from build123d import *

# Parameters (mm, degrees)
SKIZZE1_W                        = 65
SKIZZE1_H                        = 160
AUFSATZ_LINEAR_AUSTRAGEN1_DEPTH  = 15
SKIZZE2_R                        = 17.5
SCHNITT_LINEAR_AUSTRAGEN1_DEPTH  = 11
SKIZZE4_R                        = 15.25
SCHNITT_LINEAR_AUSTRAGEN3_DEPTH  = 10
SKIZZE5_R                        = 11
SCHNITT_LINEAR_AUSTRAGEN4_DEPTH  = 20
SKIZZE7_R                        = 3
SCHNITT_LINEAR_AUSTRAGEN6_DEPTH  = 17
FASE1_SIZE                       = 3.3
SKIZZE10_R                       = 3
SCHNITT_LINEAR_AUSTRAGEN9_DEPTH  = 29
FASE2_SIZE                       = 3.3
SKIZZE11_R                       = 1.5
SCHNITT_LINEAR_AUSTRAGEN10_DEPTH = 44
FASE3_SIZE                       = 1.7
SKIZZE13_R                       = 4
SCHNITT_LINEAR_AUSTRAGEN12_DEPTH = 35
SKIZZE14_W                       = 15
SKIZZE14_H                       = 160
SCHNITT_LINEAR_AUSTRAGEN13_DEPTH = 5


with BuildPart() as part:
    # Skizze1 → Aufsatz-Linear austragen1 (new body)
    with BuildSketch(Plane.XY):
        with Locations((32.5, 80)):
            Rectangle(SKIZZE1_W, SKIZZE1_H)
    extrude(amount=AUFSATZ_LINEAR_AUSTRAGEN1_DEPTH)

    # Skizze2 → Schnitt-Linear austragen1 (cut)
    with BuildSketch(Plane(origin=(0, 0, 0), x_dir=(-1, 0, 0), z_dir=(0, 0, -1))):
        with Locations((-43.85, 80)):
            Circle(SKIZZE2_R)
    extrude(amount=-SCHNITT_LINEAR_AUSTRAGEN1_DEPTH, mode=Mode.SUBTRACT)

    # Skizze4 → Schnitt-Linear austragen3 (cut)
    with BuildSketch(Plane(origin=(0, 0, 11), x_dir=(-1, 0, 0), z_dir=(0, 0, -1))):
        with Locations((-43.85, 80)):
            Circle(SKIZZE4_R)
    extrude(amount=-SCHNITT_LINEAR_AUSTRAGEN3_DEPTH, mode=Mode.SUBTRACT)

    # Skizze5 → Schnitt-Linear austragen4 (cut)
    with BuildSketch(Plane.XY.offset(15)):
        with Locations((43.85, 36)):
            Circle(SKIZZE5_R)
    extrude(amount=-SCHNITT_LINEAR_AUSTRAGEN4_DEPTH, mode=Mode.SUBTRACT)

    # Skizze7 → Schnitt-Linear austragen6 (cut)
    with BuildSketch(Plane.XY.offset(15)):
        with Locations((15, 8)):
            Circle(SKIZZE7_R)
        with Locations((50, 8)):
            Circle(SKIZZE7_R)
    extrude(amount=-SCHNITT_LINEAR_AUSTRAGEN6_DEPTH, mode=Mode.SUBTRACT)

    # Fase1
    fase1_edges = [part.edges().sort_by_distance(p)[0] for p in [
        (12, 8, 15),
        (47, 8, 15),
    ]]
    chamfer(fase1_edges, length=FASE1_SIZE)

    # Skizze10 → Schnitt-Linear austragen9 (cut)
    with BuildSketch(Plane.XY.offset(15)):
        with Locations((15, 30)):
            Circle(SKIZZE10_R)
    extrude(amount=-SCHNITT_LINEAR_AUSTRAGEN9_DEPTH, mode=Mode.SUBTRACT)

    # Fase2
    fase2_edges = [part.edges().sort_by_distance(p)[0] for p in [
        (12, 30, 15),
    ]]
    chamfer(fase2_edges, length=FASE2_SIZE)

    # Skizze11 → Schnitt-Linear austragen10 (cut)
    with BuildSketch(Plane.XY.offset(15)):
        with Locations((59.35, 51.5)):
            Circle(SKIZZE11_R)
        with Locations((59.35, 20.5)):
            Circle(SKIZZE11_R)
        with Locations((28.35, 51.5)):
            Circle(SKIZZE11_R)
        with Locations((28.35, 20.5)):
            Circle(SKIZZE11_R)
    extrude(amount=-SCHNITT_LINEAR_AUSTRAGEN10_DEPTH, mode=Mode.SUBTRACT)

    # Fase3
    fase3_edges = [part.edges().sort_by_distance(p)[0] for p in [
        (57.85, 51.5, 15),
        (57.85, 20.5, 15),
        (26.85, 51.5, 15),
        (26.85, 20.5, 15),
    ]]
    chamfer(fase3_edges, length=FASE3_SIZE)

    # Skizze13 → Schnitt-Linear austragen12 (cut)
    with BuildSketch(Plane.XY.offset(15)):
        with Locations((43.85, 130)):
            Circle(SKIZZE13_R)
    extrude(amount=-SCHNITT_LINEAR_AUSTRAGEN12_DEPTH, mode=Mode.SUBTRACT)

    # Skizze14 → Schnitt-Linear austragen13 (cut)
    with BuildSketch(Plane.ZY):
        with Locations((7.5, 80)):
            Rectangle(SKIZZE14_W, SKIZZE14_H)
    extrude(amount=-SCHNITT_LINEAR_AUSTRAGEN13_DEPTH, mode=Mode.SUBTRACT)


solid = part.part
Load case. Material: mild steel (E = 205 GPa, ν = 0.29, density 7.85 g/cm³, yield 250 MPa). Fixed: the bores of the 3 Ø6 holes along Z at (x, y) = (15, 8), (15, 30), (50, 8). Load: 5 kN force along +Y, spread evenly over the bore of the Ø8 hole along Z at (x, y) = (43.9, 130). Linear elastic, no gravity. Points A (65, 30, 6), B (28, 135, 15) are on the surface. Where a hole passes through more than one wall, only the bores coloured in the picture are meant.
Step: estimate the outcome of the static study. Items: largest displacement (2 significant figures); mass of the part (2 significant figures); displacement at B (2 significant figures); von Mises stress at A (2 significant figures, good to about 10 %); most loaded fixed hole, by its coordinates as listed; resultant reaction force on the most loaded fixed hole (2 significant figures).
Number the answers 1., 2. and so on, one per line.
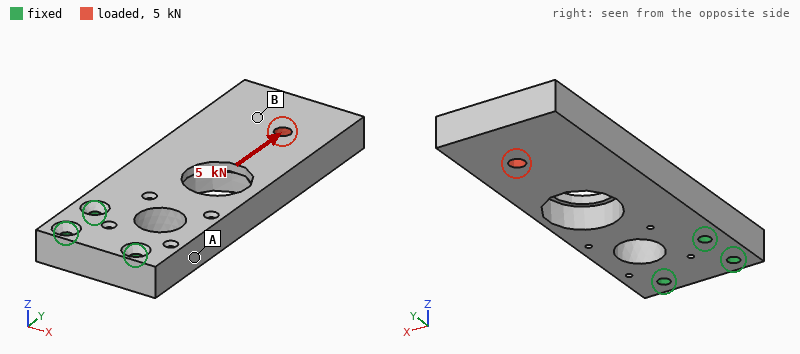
1. 29 µm
2. 960 g
3. 18 µm
4. 11 MPa
5. (50, 8)
6. 3.4 kN
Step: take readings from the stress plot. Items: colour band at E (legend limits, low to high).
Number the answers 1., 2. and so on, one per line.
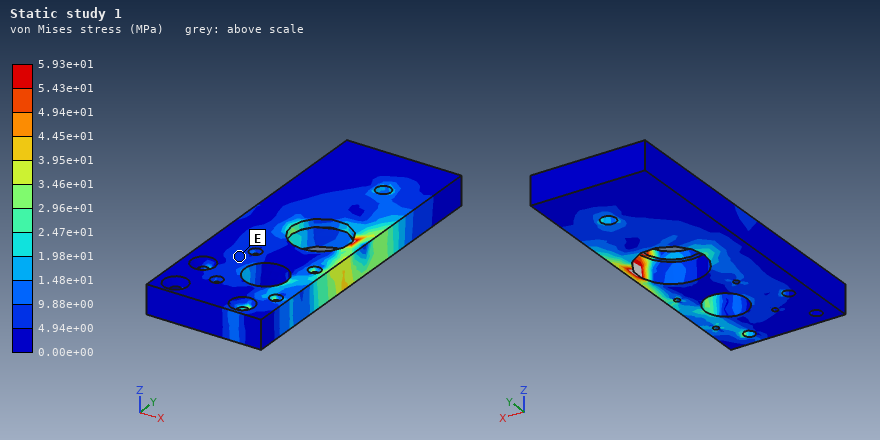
1. 4.94e+00 to 9.88e+00 MPa
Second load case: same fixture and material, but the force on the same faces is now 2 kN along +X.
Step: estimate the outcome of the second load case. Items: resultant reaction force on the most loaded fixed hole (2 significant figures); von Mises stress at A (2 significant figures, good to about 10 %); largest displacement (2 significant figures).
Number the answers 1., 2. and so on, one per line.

1. 5.0 kN
2. 19 MPa
3. 49 µm
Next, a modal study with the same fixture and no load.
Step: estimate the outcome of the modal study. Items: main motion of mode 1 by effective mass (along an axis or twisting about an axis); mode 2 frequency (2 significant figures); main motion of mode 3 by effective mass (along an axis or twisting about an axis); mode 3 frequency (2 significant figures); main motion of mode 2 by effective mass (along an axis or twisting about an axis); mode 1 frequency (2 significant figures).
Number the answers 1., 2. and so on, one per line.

1. along Z
2. 1700 Hz
3. twisting about Y
4. 2200 Hz
5. along X
6. 530 Hz
